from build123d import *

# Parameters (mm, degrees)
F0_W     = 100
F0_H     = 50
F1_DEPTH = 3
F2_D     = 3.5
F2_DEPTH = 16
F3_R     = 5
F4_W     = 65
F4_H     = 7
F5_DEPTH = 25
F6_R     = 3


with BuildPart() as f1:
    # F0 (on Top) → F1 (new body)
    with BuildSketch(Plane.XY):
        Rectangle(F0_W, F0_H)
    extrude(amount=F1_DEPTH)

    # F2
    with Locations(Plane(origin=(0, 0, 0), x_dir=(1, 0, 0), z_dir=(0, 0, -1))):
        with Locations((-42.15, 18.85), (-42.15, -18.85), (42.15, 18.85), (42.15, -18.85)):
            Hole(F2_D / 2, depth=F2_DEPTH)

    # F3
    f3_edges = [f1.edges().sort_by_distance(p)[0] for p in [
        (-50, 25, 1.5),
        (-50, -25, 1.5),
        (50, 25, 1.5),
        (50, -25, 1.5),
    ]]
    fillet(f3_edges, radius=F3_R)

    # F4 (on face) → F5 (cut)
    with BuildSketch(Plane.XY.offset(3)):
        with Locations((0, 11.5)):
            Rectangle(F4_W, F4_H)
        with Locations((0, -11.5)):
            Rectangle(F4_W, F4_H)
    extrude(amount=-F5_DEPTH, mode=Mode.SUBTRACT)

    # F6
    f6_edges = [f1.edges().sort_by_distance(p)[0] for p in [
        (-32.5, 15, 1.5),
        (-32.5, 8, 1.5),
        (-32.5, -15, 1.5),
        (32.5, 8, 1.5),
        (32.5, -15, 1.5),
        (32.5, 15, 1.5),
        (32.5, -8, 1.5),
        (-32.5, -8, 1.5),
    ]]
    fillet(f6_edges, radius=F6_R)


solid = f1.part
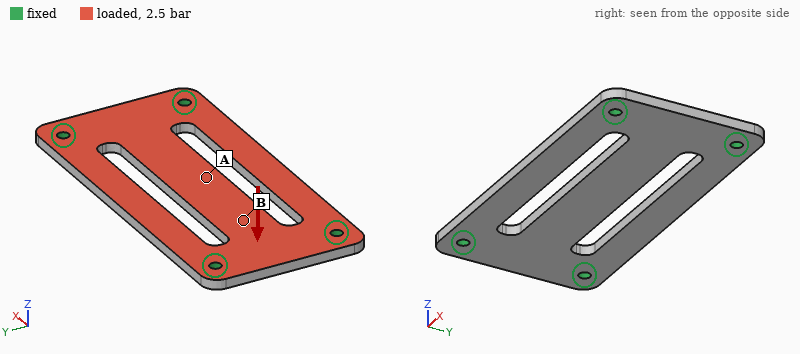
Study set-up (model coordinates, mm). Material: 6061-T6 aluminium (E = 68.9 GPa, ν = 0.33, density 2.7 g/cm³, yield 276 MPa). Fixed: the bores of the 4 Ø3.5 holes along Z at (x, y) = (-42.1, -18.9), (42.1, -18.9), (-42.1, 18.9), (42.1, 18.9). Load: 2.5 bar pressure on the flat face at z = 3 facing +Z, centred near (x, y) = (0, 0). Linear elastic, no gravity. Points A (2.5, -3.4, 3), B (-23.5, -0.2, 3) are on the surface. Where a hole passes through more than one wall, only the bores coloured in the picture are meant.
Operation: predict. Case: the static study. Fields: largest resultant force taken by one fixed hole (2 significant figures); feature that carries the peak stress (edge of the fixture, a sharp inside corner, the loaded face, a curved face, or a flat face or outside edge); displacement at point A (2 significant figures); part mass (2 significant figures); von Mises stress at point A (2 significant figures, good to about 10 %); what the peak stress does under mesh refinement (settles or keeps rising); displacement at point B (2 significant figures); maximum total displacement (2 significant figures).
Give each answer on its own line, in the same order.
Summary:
250 N
edge of the fixture
0.25 mm
33 g
50 MPa
keeps rising
0.13 mm
0.25 mm
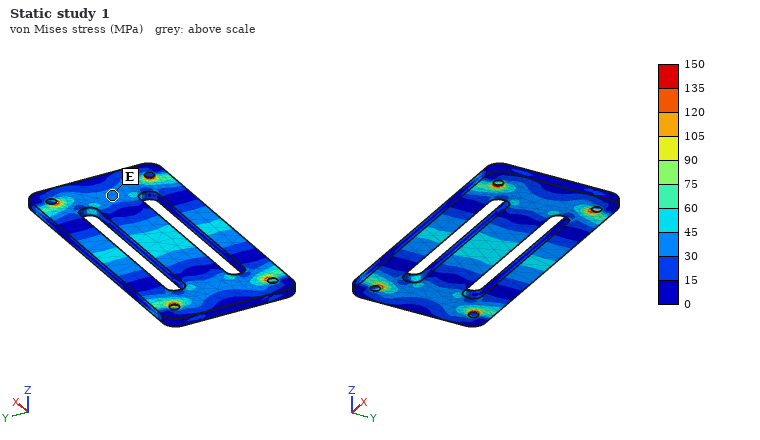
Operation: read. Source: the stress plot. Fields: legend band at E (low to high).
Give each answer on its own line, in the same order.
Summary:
30 to 45 MPa
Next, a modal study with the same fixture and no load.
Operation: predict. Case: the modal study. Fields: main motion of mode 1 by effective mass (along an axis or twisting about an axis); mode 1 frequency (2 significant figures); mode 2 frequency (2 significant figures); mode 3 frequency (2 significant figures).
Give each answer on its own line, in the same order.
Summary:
along Z
2100 Hz
2500 Hz
2600 Hz
